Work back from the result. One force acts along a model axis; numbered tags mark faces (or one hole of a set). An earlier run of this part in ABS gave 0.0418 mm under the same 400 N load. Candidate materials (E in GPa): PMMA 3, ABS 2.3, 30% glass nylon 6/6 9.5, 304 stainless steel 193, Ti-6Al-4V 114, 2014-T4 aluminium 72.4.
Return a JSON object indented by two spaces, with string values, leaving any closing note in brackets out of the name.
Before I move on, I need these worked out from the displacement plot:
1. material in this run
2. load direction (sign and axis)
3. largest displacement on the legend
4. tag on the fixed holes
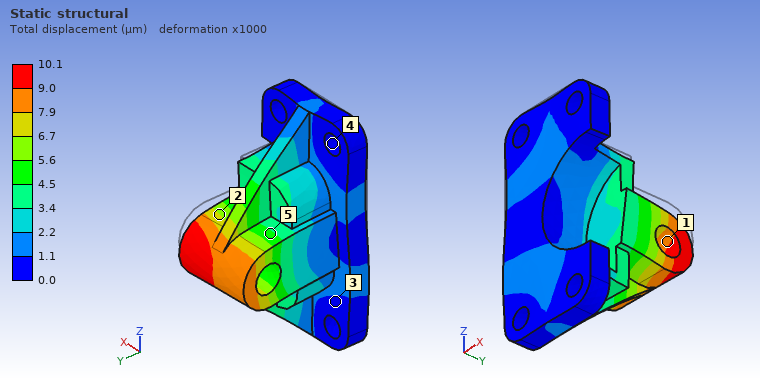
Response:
{
  "material in this run": "30% glass nylon 6/6",
  "load direction": "-Z",
  "largest displacement on the legend": "10.1 µm",
  "tag on the fixed holes": "4"
}
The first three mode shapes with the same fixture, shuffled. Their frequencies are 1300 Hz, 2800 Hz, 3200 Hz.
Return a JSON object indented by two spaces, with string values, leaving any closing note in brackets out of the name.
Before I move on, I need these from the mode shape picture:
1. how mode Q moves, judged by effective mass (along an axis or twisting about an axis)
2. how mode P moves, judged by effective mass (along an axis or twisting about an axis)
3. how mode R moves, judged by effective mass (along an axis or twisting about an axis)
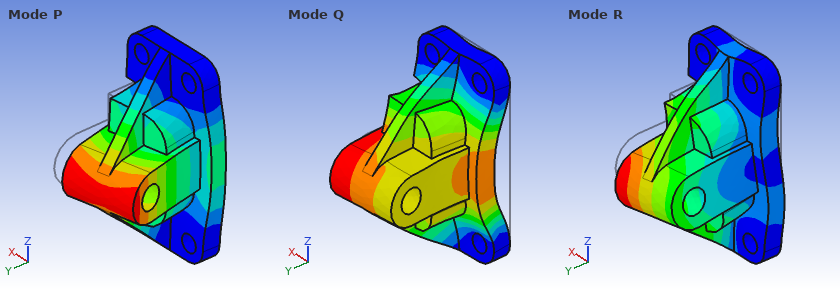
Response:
{
  "how mode Q moves, judged by effective mass": "along Y",
  "how mode P moves, judged by effective mass": "along X",
  "how mode R moves, judged by effective mass": "along Z"
}
